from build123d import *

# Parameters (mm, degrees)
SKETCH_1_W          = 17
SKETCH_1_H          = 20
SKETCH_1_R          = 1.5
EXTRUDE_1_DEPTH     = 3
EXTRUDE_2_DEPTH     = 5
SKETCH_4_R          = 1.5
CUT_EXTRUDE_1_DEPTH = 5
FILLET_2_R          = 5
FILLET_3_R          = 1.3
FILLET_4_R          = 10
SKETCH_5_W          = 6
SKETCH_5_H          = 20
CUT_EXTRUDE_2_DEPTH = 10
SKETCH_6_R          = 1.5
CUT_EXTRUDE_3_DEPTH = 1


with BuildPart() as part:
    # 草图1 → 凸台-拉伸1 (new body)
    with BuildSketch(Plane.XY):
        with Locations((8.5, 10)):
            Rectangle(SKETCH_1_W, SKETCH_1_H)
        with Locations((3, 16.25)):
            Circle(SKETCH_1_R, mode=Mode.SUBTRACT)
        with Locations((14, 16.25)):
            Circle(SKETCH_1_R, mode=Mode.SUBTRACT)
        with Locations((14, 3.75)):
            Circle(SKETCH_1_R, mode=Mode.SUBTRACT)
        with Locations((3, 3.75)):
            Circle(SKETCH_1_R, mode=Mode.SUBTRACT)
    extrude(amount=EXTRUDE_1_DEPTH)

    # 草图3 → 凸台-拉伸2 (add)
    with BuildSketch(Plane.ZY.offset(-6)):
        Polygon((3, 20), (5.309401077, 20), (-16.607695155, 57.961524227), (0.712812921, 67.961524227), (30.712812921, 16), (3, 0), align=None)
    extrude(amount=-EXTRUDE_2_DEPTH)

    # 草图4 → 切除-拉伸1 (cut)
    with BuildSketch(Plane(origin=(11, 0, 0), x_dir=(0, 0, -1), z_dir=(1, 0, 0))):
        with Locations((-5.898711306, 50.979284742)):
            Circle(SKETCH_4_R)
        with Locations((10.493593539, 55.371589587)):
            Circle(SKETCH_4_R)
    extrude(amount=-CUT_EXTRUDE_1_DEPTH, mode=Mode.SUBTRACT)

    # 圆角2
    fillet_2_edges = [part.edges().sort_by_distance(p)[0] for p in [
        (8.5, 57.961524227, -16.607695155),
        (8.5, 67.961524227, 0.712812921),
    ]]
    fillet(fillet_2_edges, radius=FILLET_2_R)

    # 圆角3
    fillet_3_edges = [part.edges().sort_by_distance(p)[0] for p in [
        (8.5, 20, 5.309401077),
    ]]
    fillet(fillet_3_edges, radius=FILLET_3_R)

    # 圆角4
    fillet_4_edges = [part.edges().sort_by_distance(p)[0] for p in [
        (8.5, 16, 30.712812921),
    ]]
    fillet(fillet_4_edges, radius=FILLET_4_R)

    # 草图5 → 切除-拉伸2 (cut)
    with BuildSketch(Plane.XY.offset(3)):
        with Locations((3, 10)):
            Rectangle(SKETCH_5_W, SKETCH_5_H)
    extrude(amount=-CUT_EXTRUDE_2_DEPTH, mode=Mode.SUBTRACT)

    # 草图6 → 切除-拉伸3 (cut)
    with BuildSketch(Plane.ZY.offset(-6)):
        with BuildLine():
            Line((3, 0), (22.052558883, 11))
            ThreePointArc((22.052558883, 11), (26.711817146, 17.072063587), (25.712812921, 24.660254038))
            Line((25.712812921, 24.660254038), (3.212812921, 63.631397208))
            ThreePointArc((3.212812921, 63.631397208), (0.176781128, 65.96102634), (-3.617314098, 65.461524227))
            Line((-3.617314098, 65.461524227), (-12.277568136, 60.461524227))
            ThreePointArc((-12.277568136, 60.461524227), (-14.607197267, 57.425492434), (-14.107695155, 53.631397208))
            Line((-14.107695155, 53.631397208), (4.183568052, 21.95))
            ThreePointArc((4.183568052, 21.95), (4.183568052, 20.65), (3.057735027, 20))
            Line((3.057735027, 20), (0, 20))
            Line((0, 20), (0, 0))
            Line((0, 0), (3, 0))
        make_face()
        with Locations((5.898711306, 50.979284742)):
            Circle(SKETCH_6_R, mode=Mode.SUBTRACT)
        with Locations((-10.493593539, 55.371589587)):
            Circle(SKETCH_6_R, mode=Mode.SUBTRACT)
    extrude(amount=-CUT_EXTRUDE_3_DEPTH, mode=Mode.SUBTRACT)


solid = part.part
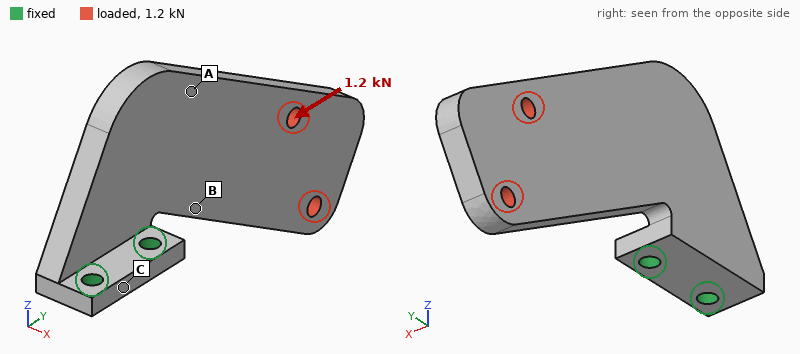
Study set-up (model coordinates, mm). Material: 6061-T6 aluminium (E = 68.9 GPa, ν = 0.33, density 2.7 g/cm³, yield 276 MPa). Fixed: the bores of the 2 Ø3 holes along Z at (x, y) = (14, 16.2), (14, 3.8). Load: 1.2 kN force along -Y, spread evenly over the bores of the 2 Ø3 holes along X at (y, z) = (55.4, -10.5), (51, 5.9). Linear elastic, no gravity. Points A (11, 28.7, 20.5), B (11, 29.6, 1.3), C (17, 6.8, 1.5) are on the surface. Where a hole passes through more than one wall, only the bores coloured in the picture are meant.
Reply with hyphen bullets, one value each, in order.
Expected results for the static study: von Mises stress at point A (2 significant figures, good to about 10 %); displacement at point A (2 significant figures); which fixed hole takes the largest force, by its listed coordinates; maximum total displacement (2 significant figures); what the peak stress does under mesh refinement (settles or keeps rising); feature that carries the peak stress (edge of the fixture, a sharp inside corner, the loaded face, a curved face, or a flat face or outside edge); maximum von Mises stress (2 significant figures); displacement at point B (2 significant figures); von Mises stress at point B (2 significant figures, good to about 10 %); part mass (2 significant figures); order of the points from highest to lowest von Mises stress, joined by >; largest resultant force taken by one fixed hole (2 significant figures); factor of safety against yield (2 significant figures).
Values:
- 30 MPa
- 0.052 mm
- (14, 16.2)
- 0.21 mm
- settles
- a curved face
- 310 MPa
- 0.053 mm
- 56 MPa
- 15 g
- B > A > C
- 870 N
- 0.90
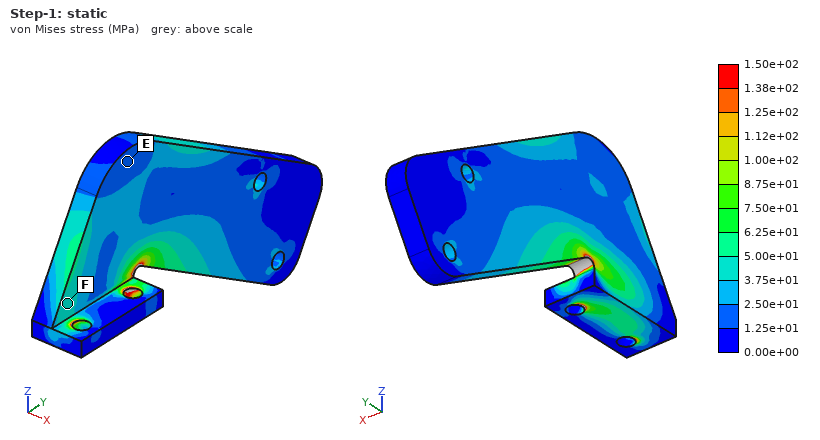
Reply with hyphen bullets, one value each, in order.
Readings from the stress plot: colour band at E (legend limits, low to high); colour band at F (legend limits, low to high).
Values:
- 1.25e+01 to 2.50e+01 MPa
- 3.75e+01 to 5.00e+01 MPa
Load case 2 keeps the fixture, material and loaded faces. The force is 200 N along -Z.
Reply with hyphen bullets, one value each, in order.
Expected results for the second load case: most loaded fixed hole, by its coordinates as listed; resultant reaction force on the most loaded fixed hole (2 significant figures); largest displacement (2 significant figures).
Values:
- (14, 16.2)
- 710 N
- 0.17 mm
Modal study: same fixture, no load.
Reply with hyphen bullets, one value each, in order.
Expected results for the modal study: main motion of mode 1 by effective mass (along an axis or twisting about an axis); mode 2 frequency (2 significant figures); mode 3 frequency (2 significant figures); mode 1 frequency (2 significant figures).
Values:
- along X
- 2300 Hz
- 2900 Hz
- 1100 Hz
